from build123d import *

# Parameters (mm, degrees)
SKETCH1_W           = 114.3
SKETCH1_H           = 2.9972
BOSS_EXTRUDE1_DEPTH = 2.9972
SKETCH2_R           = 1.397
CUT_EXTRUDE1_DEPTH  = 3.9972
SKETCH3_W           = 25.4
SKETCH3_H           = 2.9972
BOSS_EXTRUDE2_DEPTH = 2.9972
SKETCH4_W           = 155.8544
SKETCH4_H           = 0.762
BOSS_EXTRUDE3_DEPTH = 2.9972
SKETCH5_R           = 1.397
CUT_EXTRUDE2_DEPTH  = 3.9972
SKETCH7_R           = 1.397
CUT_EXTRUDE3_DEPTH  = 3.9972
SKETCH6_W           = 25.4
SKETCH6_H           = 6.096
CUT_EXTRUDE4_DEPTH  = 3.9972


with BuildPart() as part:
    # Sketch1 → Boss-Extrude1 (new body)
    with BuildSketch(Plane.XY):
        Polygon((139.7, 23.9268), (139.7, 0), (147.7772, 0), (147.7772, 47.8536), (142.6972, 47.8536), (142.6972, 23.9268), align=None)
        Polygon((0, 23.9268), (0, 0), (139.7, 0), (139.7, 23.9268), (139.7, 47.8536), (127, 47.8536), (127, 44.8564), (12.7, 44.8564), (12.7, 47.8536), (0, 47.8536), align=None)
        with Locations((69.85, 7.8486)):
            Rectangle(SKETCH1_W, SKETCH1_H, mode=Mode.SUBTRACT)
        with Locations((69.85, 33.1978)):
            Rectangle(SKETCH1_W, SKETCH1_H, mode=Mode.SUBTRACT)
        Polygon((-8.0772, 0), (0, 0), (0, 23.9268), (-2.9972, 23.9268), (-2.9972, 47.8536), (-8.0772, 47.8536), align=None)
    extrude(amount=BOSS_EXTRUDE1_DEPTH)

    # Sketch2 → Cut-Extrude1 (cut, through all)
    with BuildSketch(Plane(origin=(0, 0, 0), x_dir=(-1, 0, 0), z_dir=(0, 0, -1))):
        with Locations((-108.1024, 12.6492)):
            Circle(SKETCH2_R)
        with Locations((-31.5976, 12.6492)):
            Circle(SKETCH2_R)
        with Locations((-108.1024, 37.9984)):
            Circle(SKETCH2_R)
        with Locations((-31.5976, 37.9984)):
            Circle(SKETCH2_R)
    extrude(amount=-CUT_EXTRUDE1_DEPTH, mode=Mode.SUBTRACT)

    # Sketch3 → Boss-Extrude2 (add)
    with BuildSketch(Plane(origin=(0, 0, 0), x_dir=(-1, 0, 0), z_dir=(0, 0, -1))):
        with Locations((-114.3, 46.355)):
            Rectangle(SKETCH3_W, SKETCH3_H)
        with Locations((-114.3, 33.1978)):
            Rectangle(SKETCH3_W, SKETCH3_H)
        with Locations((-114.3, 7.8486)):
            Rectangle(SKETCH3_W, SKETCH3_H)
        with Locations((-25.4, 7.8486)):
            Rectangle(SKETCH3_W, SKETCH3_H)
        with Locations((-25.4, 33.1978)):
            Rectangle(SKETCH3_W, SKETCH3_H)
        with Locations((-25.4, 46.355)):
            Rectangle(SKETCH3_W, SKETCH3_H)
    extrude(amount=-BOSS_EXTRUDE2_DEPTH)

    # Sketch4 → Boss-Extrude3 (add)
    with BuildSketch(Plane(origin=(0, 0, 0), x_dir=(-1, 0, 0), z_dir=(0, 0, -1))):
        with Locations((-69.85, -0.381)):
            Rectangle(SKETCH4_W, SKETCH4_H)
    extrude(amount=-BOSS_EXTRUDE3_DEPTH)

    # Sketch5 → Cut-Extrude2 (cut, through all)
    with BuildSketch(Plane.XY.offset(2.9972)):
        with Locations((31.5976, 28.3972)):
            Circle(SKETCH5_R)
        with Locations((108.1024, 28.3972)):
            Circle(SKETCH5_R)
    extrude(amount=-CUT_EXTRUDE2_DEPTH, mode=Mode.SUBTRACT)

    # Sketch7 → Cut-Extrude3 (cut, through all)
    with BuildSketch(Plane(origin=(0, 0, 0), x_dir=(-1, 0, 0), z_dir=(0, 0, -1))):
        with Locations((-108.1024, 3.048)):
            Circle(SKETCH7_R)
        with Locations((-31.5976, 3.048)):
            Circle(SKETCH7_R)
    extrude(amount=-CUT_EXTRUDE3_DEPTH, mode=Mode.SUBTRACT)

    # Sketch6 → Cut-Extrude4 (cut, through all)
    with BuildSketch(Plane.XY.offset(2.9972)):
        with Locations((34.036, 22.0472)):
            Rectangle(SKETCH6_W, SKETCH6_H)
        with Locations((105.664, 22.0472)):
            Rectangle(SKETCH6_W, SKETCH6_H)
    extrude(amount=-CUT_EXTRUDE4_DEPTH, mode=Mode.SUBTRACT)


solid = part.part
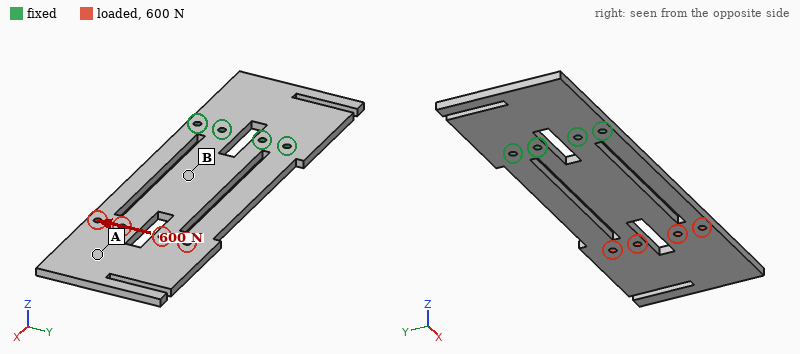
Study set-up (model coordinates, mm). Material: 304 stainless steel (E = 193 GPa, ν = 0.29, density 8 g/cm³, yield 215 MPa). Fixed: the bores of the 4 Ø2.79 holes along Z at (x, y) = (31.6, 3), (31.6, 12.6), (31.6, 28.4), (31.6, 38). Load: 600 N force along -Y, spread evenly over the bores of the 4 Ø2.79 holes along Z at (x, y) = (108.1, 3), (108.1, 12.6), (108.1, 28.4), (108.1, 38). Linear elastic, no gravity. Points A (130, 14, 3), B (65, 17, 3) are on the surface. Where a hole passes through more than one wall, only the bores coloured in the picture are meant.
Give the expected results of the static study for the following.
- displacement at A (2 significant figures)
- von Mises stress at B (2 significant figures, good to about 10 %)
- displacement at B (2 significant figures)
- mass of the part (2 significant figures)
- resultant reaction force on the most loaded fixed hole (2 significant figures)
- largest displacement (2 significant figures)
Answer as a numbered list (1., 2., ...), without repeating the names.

1. 70 µm
2. 20 MPa
3. 21 µm
4. 160 g
5. 1.0 kN
6. 79 µm
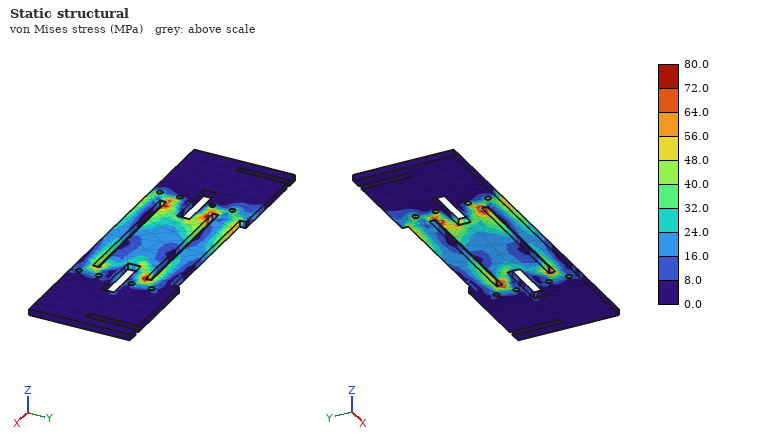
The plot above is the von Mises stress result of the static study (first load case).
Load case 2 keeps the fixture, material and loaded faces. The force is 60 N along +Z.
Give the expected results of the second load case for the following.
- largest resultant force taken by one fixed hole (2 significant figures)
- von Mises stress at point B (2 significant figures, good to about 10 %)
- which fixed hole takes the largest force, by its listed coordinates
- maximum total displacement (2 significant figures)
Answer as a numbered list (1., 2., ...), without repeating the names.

1. 28 N
2. 40 MPa
3. (31.6, 12.6)
4. 0.98 mm
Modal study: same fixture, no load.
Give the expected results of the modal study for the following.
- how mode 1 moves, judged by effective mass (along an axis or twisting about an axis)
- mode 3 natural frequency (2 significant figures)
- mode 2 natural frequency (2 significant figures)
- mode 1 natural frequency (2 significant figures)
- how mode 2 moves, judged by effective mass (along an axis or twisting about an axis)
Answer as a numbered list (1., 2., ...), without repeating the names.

1. along Z
2. 1100 Hz
3. 790 Hz
4. 160 Hz
5. twisting about X
